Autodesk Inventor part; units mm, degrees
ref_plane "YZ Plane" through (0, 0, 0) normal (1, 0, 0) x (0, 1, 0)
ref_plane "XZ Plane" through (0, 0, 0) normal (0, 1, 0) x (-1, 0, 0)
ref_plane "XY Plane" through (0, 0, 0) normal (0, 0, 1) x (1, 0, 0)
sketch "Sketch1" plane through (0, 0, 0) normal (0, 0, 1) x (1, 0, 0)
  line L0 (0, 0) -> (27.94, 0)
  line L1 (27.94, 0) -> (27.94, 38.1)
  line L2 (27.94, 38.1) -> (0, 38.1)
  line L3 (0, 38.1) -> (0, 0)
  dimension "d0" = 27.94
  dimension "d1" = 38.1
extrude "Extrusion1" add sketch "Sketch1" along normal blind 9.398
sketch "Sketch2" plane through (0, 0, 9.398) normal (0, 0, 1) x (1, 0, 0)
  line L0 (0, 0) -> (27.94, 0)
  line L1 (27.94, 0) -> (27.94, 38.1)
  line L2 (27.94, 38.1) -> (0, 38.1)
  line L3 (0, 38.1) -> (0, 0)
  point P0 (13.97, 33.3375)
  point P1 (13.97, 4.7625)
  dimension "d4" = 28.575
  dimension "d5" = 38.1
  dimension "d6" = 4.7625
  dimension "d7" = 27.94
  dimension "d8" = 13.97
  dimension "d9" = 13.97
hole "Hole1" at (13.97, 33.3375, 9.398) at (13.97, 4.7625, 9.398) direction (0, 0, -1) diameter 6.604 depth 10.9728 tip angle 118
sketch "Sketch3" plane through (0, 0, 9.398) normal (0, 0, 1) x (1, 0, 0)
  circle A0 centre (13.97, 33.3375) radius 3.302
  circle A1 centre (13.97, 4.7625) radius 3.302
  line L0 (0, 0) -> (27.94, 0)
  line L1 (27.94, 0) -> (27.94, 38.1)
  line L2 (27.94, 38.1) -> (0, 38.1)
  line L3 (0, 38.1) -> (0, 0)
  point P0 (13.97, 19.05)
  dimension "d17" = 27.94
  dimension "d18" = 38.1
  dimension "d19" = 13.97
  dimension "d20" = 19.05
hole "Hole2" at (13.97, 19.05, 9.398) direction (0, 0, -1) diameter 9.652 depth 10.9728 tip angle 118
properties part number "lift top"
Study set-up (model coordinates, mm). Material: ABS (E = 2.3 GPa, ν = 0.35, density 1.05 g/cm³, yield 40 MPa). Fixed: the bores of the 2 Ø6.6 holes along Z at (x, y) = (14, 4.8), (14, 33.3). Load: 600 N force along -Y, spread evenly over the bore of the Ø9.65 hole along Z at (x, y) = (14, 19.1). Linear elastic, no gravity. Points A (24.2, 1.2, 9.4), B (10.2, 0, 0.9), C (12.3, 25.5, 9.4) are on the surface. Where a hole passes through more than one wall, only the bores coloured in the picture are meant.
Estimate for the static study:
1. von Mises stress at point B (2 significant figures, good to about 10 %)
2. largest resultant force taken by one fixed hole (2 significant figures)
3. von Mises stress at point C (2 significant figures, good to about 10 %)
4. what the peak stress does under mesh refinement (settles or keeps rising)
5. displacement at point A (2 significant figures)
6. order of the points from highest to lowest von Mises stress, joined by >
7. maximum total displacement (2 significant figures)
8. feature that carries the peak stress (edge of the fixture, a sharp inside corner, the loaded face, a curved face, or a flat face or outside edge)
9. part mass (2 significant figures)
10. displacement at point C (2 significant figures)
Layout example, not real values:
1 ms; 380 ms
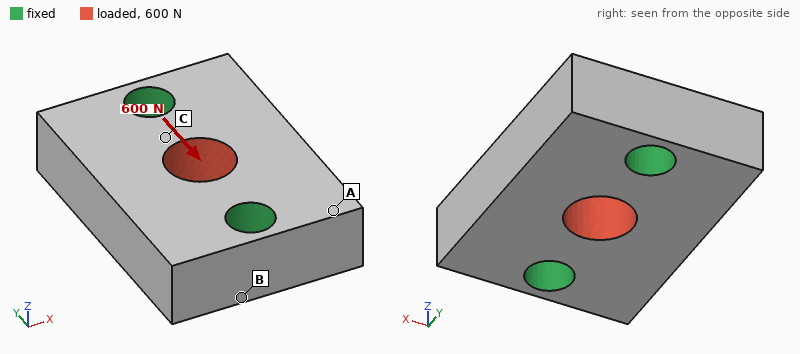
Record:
0.79 MPa; 300 N; 2.9 MPa; keeps rising; 5.8 µm; C > B > A; 13 µm; edge of the fixture; 9.1 g; 6.4 µm
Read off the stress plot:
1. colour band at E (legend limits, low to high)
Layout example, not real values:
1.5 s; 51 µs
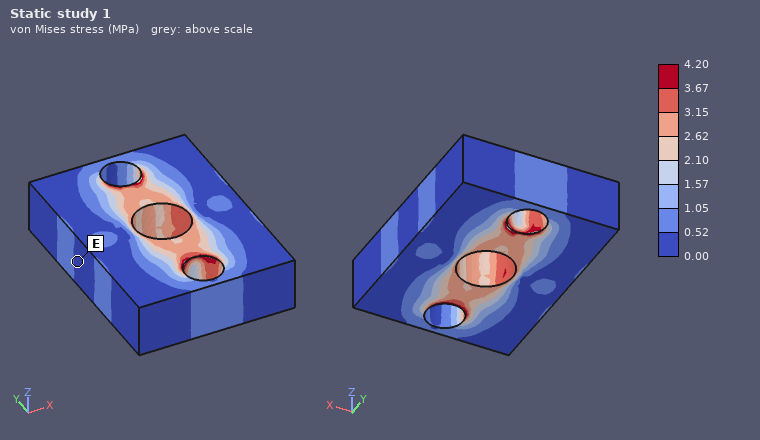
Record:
0.00 to 0.52 MPa
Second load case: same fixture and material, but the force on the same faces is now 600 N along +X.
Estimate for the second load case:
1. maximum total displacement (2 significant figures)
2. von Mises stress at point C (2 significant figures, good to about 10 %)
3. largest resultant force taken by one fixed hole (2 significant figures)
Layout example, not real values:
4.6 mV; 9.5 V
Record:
23 µm; 2.9 MPa; 300 N
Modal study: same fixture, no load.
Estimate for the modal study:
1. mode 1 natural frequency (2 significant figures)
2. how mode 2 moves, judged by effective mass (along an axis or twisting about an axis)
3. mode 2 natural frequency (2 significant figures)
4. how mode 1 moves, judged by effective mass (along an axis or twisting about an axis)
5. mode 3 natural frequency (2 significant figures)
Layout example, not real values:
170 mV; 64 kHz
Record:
8200 Hz; along Z; 9000 Hz; twisting about Y; 12 kHz
